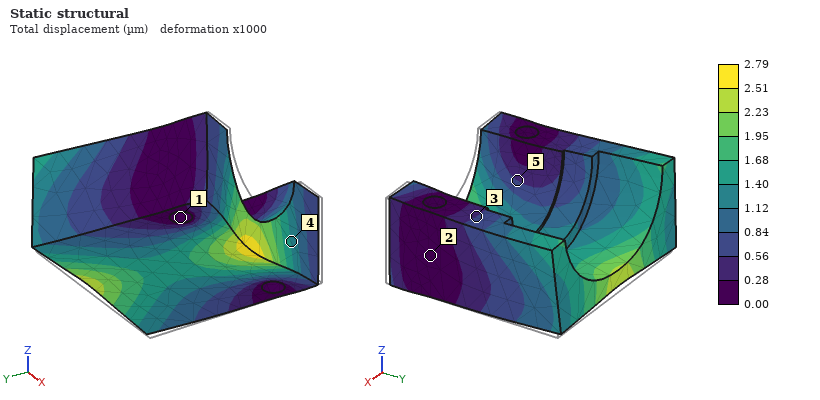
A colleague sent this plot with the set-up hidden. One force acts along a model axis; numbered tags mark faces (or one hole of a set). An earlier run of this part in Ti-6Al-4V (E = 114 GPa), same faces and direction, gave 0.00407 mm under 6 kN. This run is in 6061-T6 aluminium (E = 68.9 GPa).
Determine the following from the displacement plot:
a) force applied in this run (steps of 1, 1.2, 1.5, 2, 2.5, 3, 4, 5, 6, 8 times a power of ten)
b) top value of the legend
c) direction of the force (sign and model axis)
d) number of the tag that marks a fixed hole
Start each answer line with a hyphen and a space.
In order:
- 2.5 kN
- 2.79 µm
- +Y
- 1
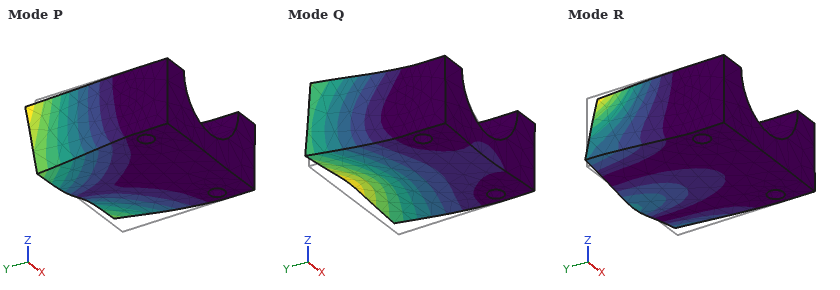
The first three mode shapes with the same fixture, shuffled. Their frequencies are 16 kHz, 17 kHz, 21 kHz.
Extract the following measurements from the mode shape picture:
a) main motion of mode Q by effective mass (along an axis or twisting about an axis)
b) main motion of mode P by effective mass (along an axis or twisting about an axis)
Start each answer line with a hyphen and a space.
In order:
- along Z
- along X
